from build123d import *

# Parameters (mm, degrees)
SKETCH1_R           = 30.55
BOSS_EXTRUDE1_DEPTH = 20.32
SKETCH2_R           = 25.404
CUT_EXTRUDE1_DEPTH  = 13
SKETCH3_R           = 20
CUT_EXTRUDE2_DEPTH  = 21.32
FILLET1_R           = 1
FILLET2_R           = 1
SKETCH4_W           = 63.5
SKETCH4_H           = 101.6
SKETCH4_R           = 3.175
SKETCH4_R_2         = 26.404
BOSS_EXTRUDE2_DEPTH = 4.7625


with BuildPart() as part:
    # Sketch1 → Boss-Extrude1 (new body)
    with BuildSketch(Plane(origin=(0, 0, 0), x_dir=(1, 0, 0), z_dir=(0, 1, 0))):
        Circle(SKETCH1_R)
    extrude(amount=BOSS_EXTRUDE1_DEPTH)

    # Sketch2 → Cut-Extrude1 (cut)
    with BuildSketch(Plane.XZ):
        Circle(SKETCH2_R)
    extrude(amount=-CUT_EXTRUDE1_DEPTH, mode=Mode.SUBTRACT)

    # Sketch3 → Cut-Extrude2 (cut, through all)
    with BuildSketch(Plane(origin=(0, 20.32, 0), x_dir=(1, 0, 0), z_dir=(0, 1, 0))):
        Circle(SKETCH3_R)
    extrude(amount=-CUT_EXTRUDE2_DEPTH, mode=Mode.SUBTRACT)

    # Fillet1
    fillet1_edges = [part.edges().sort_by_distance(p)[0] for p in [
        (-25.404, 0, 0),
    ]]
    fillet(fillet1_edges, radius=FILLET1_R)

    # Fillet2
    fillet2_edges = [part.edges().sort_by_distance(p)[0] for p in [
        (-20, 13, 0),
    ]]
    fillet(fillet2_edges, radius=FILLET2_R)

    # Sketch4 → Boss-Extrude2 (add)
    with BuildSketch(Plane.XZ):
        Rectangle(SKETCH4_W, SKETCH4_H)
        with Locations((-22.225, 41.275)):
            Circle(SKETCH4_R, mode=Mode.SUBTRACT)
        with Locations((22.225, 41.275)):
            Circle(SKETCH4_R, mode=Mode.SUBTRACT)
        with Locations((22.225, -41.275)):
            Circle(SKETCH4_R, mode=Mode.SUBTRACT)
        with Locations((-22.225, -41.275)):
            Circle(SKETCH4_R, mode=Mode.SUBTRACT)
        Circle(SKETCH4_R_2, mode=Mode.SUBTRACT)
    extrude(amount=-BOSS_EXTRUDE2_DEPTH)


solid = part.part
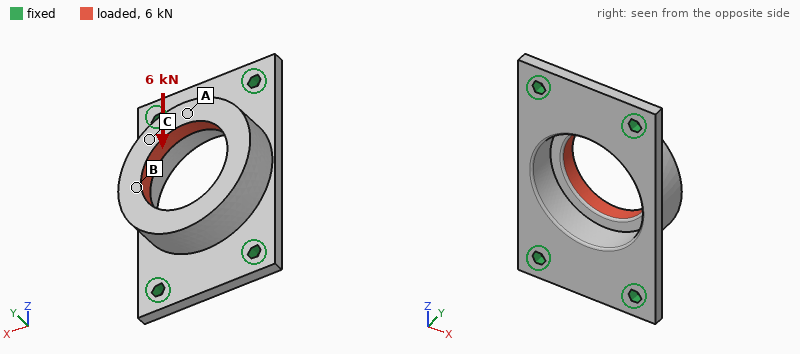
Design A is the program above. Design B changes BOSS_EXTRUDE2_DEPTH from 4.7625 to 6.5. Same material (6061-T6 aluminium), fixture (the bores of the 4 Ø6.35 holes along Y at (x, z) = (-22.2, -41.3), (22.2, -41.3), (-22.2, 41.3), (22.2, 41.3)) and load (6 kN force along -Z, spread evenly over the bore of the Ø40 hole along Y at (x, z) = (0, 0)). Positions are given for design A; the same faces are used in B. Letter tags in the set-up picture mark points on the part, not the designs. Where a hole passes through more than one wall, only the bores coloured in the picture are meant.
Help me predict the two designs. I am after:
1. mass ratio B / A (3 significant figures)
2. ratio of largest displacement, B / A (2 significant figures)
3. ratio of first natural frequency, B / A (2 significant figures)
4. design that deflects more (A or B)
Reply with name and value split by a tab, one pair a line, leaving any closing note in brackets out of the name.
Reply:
mass ratio B / A	1.15
ratio of largest displacement, B / A	0.62
ratio of first natural frequency, B / A	1.3
design that deflects more	A
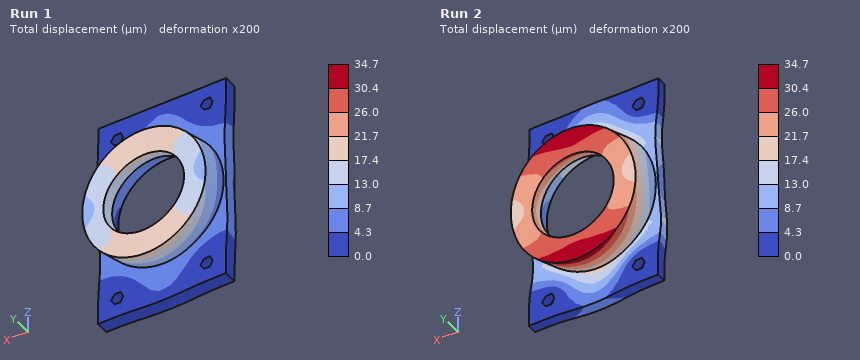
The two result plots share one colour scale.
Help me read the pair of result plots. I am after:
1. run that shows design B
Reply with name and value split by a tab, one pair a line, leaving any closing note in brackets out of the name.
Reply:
run that shows design B	Run 1
